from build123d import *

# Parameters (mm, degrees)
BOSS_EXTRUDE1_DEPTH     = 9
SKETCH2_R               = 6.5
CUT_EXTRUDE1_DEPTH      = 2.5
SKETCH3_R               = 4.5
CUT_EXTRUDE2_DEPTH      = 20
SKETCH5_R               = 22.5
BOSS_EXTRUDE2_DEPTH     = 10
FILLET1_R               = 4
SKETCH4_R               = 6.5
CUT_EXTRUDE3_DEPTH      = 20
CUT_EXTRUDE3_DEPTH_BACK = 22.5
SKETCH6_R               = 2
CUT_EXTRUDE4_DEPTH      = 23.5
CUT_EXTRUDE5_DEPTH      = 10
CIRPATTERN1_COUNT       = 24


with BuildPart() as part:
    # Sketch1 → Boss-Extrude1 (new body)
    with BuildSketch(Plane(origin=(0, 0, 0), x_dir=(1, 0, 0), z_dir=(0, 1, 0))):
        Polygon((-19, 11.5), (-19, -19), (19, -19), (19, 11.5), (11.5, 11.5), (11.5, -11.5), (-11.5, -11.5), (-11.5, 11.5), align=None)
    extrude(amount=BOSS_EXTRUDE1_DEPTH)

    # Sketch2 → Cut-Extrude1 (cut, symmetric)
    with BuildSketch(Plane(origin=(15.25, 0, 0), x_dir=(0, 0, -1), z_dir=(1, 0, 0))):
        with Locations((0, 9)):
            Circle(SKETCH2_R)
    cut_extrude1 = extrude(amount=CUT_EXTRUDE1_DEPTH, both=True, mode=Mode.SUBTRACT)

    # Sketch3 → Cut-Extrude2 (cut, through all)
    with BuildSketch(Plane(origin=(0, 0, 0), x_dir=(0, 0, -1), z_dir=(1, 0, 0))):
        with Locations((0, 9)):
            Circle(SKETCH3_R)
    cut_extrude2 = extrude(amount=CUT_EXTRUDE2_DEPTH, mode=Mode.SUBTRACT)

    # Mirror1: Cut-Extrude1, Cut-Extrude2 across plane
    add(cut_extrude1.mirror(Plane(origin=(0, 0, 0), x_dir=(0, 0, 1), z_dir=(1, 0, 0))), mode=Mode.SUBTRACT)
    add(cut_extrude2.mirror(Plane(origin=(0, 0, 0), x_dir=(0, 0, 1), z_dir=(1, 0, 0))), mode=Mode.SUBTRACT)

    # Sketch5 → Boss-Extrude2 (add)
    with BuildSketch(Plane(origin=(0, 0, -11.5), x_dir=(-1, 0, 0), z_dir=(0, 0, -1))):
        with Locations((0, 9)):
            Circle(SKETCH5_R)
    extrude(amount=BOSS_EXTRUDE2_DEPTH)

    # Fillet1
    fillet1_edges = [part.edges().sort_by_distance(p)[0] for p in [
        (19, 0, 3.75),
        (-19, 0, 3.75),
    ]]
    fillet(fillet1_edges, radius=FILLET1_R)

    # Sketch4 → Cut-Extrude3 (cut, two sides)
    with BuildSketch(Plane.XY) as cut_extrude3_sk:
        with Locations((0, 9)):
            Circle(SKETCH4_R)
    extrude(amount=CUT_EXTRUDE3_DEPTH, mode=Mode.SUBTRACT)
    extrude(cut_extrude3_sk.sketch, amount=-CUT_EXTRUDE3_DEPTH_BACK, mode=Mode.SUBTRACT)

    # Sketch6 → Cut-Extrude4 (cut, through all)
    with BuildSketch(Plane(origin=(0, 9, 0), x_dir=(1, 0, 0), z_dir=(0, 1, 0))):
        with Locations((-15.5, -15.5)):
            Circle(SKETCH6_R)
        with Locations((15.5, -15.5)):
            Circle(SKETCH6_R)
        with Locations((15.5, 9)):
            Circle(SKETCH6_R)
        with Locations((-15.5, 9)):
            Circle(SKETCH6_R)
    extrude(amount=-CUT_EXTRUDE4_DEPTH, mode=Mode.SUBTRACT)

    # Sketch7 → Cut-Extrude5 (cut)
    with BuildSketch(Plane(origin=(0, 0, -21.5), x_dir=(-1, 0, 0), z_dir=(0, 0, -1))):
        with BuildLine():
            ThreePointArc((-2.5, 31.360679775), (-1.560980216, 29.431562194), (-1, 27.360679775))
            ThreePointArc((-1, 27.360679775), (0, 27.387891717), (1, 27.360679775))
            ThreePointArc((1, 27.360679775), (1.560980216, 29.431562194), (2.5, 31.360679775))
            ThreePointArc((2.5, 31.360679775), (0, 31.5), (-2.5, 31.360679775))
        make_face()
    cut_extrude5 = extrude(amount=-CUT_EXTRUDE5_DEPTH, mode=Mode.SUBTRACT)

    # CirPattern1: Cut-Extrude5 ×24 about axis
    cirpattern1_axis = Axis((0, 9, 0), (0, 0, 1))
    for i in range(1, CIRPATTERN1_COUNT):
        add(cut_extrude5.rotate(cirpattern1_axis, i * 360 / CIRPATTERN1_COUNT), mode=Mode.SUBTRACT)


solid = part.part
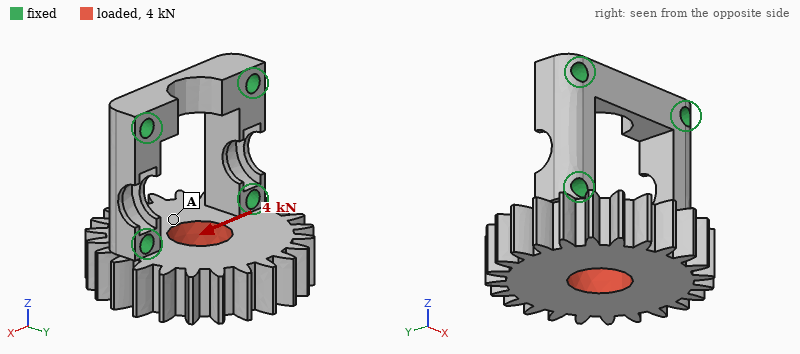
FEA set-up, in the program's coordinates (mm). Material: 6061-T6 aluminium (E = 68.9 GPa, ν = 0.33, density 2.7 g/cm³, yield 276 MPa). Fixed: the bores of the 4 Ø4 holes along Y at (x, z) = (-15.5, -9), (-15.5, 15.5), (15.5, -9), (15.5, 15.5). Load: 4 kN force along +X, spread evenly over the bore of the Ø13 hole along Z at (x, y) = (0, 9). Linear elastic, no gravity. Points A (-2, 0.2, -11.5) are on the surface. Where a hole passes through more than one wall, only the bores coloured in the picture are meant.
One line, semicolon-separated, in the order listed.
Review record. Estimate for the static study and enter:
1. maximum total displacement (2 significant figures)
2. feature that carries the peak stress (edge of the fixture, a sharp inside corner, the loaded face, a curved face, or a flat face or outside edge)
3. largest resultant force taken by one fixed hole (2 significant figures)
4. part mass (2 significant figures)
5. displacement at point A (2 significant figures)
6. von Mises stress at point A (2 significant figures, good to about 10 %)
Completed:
13 µm; edge of the fixture; 2.2 kN; 41 g; 6.6 µm; 16 MPa
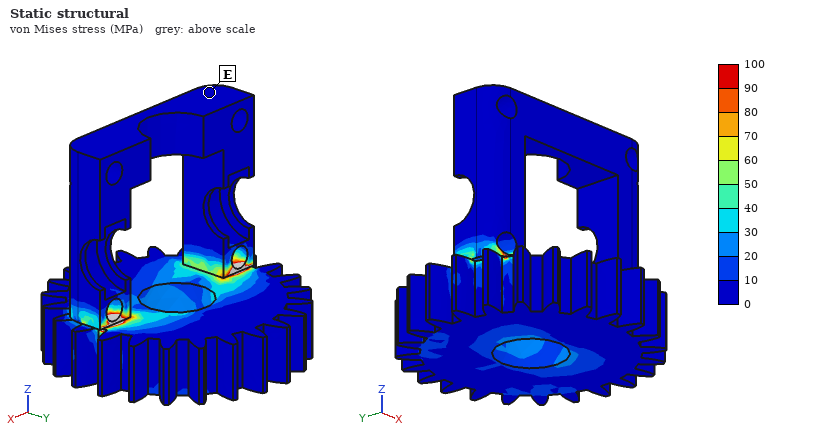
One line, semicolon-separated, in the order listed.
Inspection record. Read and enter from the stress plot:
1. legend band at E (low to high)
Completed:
0 to 10 MPa
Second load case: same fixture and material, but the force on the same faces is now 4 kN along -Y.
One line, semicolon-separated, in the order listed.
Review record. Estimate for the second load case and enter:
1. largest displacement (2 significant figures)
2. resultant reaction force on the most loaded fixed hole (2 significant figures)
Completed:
50 µm; 2.0 kN
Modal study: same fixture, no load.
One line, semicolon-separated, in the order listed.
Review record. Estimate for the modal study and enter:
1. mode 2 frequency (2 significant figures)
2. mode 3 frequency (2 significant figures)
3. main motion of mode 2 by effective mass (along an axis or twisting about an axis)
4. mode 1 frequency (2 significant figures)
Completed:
16 kHz; 18 kHz; along X; 7200 Hz
